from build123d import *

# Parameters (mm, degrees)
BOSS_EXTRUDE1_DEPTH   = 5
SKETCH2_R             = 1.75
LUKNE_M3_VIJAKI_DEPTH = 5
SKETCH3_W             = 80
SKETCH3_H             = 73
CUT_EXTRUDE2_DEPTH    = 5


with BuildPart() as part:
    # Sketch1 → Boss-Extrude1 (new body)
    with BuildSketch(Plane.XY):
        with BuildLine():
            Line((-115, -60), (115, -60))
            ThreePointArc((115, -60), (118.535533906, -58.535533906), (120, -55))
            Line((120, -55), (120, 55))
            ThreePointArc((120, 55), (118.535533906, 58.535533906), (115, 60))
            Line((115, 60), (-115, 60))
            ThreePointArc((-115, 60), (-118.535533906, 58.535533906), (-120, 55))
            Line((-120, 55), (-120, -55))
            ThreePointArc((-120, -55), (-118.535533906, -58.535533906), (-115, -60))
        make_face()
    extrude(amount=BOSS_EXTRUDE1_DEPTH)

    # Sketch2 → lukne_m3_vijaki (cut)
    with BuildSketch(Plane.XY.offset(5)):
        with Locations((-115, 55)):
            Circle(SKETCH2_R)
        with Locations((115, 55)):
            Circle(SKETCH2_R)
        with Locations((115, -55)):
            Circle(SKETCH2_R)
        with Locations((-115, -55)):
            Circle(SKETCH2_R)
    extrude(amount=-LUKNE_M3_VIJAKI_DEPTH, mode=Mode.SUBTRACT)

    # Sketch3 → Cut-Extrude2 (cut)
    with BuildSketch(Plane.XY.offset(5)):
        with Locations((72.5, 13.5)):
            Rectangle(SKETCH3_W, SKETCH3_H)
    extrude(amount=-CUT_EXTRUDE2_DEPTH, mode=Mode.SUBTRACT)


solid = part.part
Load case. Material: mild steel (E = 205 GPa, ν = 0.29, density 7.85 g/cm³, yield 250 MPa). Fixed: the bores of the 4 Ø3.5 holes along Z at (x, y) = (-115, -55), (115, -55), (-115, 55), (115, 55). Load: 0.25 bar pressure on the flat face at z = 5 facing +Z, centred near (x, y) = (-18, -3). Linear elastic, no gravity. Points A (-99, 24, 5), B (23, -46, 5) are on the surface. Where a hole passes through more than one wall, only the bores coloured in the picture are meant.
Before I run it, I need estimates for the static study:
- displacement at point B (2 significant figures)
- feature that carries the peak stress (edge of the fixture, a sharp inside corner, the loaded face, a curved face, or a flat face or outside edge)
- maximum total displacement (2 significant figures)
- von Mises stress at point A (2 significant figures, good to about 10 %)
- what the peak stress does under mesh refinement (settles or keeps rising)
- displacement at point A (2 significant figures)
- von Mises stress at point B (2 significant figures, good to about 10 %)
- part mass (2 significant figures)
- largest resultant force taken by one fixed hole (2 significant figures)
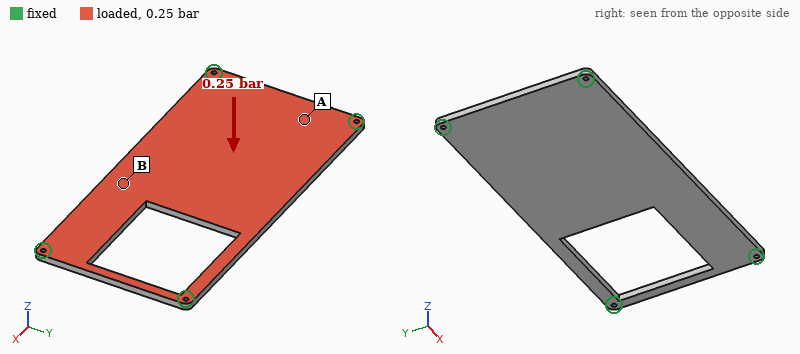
0.14 mm
edge of the fixture
0.17 mm
8.6 MPa
keeps rising
0.029 mm
21 MPa
900 g
180 N
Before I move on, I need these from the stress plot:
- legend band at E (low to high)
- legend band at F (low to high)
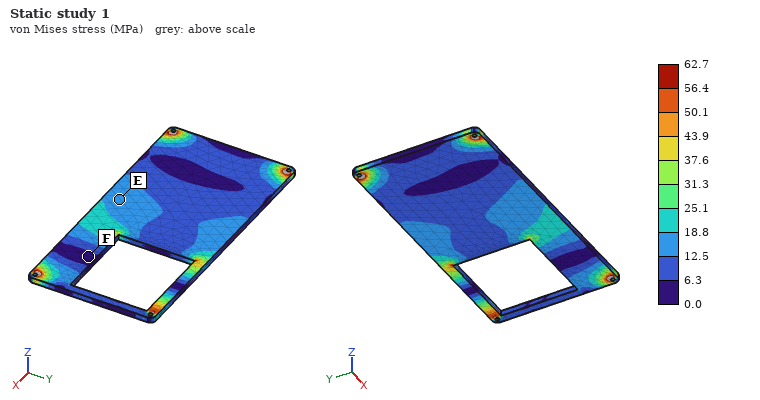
12.5 to 18.8 MPa
0.0 to 6.3 MPa
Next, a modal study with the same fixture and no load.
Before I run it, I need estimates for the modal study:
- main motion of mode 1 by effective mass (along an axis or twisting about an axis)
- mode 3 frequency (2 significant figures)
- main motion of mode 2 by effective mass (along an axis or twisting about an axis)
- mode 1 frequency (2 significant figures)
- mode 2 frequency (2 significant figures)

along Z
1100 Hz
twisting about X
350 Hz
670 Hz
